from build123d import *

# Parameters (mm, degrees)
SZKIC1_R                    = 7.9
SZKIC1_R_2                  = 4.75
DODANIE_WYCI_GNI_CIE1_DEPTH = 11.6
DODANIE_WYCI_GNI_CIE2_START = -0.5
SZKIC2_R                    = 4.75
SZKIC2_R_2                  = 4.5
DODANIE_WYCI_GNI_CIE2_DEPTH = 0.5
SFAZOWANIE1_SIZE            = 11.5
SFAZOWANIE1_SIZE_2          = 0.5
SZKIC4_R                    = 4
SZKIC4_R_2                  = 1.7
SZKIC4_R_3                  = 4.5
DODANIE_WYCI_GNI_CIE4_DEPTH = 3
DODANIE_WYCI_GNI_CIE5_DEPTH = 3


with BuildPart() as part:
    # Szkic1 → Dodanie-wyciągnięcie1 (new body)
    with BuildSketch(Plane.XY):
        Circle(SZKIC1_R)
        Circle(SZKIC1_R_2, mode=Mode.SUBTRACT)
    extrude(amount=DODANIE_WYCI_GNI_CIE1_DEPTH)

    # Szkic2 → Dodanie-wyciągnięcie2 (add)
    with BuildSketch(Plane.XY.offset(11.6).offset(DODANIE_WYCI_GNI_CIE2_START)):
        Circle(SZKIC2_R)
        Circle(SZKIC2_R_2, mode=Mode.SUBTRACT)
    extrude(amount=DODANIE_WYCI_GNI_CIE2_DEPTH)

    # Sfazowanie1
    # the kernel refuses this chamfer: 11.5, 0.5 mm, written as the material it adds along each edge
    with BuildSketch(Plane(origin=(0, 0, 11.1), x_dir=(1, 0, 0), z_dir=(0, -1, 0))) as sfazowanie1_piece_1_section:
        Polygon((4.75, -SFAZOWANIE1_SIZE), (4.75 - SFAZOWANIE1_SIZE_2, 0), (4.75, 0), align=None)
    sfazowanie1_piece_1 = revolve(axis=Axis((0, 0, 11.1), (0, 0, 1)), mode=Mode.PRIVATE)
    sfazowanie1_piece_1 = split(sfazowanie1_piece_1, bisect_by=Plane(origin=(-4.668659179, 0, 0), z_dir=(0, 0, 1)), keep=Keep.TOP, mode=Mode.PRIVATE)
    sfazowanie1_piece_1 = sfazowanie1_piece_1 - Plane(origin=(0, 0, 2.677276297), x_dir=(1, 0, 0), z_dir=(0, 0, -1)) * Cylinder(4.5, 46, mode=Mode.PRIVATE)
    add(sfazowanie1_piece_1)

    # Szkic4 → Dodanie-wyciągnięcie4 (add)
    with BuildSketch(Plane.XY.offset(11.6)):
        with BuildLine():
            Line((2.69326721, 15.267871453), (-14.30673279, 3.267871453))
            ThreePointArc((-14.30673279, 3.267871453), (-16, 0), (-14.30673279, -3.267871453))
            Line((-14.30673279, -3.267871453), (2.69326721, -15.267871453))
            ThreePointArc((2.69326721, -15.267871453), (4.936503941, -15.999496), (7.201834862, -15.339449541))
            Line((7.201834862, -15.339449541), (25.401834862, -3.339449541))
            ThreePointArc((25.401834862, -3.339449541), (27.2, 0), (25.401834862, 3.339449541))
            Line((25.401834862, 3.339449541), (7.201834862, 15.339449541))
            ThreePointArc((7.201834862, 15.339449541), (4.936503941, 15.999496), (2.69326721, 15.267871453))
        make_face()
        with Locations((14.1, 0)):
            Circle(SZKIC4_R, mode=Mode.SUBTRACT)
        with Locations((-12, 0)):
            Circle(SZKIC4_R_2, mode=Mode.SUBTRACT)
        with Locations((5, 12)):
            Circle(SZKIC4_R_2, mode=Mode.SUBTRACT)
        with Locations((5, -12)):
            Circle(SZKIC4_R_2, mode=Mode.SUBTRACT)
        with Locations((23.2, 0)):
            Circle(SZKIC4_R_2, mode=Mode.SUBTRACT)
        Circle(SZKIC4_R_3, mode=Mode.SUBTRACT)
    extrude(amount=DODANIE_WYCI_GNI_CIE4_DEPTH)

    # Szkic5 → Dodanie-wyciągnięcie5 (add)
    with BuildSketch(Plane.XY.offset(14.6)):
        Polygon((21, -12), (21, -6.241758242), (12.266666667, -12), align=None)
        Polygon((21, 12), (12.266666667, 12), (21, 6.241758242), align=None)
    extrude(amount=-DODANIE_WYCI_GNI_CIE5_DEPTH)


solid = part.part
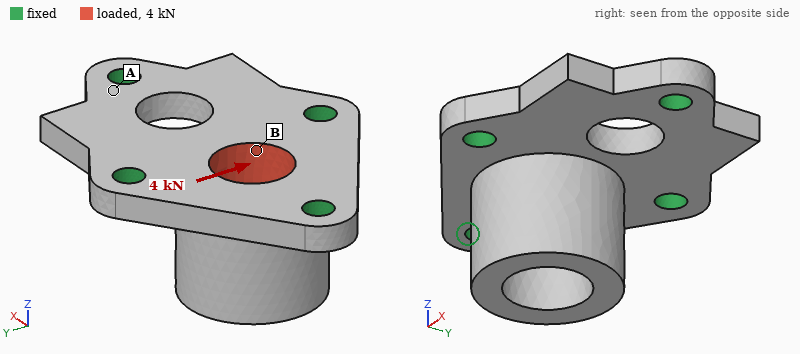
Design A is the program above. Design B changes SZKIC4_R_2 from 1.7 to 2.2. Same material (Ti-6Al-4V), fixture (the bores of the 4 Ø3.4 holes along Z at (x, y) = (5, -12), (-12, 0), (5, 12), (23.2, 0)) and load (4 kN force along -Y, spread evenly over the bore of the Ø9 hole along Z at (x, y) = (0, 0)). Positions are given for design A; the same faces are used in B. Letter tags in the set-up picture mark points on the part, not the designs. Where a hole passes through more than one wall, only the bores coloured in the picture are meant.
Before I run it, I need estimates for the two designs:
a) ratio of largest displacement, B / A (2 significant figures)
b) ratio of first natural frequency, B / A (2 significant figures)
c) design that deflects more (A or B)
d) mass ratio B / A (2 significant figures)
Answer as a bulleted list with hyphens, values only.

- 0.85
- 1.1
- A
- 0.98
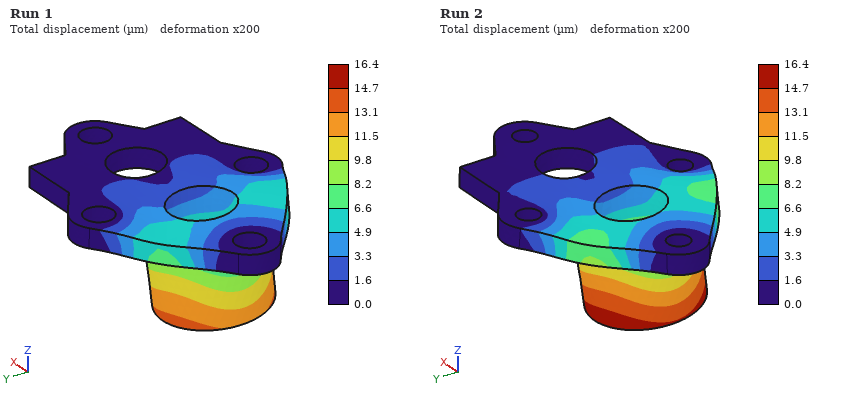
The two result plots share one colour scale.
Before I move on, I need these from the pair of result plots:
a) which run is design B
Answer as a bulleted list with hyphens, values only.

- Run 1
